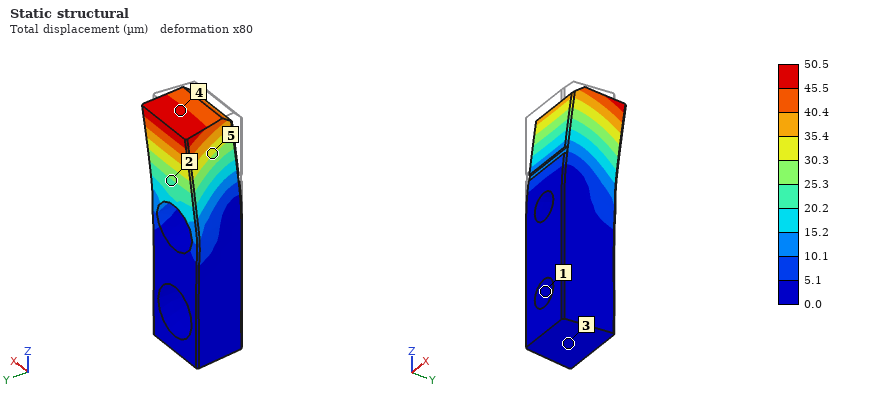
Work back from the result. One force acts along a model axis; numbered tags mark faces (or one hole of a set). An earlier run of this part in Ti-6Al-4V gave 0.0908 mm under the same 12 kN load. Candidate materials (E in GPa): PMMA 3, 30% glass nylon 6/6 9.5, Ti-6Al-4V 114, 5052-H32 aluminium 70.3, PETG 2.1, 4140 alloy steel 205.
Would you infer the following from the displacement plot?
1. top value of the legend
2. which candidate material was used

50.5 µm
4140 alloy steel
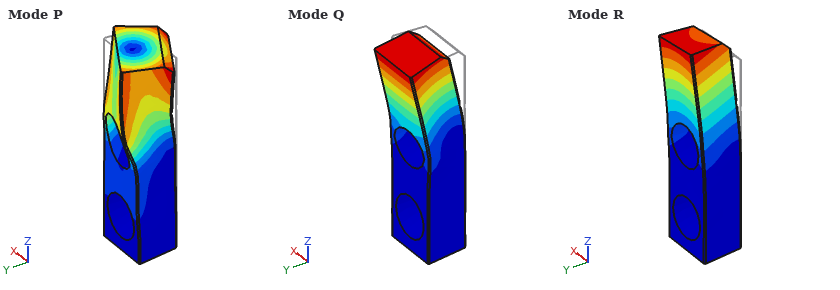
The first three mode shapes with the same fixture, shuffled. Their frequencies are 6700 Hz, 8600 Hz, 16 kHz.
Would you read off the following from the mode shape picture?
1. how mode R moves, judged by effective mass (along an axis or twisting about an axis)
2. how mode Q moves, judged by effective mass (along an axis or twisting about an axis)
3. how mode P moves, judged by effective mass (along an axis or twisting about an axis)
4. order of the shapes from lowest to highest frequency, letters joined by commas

along X
along Y
twisting about Z
Q, R, P
